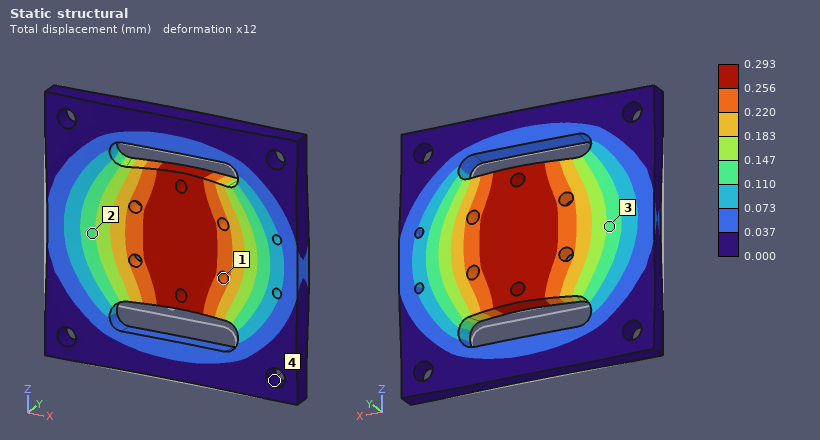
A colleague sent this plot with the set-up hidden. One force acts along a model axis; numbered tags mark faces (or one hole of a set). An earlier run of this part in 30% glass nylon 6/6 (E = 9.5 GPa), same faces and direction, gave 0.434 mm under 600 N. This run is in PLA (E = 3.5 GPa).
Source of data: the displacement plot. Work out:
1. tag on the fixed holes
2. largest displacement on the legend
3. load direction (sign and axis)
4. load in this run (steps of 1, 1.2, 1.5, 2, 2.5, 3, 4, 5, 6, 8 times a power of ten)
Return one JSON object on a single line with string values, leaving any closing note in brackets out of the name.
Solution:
{"tag on the fixed holes": "4", "largest displacement on the legend": "0.293 mm", "load direction": "+Y", "load in this run": "150 N"}
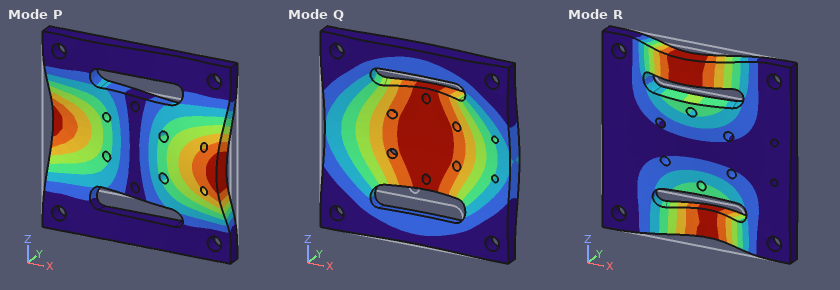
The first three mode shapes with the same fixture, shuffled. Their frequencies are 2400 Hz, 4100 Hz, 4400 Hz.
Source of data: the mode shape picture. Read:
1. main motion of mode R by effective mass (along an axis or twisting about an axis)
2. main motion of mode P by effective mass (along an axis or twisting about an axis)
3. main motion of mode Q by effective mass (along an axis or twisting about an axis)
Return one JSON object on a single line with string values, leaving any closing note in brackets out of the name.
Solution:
{"main motion of mode R by effective mass": "twisting about X", "main motion of mode P by effective mass": "twisting about Z", "main motion of mode Q by effective mass": "along Y"}
